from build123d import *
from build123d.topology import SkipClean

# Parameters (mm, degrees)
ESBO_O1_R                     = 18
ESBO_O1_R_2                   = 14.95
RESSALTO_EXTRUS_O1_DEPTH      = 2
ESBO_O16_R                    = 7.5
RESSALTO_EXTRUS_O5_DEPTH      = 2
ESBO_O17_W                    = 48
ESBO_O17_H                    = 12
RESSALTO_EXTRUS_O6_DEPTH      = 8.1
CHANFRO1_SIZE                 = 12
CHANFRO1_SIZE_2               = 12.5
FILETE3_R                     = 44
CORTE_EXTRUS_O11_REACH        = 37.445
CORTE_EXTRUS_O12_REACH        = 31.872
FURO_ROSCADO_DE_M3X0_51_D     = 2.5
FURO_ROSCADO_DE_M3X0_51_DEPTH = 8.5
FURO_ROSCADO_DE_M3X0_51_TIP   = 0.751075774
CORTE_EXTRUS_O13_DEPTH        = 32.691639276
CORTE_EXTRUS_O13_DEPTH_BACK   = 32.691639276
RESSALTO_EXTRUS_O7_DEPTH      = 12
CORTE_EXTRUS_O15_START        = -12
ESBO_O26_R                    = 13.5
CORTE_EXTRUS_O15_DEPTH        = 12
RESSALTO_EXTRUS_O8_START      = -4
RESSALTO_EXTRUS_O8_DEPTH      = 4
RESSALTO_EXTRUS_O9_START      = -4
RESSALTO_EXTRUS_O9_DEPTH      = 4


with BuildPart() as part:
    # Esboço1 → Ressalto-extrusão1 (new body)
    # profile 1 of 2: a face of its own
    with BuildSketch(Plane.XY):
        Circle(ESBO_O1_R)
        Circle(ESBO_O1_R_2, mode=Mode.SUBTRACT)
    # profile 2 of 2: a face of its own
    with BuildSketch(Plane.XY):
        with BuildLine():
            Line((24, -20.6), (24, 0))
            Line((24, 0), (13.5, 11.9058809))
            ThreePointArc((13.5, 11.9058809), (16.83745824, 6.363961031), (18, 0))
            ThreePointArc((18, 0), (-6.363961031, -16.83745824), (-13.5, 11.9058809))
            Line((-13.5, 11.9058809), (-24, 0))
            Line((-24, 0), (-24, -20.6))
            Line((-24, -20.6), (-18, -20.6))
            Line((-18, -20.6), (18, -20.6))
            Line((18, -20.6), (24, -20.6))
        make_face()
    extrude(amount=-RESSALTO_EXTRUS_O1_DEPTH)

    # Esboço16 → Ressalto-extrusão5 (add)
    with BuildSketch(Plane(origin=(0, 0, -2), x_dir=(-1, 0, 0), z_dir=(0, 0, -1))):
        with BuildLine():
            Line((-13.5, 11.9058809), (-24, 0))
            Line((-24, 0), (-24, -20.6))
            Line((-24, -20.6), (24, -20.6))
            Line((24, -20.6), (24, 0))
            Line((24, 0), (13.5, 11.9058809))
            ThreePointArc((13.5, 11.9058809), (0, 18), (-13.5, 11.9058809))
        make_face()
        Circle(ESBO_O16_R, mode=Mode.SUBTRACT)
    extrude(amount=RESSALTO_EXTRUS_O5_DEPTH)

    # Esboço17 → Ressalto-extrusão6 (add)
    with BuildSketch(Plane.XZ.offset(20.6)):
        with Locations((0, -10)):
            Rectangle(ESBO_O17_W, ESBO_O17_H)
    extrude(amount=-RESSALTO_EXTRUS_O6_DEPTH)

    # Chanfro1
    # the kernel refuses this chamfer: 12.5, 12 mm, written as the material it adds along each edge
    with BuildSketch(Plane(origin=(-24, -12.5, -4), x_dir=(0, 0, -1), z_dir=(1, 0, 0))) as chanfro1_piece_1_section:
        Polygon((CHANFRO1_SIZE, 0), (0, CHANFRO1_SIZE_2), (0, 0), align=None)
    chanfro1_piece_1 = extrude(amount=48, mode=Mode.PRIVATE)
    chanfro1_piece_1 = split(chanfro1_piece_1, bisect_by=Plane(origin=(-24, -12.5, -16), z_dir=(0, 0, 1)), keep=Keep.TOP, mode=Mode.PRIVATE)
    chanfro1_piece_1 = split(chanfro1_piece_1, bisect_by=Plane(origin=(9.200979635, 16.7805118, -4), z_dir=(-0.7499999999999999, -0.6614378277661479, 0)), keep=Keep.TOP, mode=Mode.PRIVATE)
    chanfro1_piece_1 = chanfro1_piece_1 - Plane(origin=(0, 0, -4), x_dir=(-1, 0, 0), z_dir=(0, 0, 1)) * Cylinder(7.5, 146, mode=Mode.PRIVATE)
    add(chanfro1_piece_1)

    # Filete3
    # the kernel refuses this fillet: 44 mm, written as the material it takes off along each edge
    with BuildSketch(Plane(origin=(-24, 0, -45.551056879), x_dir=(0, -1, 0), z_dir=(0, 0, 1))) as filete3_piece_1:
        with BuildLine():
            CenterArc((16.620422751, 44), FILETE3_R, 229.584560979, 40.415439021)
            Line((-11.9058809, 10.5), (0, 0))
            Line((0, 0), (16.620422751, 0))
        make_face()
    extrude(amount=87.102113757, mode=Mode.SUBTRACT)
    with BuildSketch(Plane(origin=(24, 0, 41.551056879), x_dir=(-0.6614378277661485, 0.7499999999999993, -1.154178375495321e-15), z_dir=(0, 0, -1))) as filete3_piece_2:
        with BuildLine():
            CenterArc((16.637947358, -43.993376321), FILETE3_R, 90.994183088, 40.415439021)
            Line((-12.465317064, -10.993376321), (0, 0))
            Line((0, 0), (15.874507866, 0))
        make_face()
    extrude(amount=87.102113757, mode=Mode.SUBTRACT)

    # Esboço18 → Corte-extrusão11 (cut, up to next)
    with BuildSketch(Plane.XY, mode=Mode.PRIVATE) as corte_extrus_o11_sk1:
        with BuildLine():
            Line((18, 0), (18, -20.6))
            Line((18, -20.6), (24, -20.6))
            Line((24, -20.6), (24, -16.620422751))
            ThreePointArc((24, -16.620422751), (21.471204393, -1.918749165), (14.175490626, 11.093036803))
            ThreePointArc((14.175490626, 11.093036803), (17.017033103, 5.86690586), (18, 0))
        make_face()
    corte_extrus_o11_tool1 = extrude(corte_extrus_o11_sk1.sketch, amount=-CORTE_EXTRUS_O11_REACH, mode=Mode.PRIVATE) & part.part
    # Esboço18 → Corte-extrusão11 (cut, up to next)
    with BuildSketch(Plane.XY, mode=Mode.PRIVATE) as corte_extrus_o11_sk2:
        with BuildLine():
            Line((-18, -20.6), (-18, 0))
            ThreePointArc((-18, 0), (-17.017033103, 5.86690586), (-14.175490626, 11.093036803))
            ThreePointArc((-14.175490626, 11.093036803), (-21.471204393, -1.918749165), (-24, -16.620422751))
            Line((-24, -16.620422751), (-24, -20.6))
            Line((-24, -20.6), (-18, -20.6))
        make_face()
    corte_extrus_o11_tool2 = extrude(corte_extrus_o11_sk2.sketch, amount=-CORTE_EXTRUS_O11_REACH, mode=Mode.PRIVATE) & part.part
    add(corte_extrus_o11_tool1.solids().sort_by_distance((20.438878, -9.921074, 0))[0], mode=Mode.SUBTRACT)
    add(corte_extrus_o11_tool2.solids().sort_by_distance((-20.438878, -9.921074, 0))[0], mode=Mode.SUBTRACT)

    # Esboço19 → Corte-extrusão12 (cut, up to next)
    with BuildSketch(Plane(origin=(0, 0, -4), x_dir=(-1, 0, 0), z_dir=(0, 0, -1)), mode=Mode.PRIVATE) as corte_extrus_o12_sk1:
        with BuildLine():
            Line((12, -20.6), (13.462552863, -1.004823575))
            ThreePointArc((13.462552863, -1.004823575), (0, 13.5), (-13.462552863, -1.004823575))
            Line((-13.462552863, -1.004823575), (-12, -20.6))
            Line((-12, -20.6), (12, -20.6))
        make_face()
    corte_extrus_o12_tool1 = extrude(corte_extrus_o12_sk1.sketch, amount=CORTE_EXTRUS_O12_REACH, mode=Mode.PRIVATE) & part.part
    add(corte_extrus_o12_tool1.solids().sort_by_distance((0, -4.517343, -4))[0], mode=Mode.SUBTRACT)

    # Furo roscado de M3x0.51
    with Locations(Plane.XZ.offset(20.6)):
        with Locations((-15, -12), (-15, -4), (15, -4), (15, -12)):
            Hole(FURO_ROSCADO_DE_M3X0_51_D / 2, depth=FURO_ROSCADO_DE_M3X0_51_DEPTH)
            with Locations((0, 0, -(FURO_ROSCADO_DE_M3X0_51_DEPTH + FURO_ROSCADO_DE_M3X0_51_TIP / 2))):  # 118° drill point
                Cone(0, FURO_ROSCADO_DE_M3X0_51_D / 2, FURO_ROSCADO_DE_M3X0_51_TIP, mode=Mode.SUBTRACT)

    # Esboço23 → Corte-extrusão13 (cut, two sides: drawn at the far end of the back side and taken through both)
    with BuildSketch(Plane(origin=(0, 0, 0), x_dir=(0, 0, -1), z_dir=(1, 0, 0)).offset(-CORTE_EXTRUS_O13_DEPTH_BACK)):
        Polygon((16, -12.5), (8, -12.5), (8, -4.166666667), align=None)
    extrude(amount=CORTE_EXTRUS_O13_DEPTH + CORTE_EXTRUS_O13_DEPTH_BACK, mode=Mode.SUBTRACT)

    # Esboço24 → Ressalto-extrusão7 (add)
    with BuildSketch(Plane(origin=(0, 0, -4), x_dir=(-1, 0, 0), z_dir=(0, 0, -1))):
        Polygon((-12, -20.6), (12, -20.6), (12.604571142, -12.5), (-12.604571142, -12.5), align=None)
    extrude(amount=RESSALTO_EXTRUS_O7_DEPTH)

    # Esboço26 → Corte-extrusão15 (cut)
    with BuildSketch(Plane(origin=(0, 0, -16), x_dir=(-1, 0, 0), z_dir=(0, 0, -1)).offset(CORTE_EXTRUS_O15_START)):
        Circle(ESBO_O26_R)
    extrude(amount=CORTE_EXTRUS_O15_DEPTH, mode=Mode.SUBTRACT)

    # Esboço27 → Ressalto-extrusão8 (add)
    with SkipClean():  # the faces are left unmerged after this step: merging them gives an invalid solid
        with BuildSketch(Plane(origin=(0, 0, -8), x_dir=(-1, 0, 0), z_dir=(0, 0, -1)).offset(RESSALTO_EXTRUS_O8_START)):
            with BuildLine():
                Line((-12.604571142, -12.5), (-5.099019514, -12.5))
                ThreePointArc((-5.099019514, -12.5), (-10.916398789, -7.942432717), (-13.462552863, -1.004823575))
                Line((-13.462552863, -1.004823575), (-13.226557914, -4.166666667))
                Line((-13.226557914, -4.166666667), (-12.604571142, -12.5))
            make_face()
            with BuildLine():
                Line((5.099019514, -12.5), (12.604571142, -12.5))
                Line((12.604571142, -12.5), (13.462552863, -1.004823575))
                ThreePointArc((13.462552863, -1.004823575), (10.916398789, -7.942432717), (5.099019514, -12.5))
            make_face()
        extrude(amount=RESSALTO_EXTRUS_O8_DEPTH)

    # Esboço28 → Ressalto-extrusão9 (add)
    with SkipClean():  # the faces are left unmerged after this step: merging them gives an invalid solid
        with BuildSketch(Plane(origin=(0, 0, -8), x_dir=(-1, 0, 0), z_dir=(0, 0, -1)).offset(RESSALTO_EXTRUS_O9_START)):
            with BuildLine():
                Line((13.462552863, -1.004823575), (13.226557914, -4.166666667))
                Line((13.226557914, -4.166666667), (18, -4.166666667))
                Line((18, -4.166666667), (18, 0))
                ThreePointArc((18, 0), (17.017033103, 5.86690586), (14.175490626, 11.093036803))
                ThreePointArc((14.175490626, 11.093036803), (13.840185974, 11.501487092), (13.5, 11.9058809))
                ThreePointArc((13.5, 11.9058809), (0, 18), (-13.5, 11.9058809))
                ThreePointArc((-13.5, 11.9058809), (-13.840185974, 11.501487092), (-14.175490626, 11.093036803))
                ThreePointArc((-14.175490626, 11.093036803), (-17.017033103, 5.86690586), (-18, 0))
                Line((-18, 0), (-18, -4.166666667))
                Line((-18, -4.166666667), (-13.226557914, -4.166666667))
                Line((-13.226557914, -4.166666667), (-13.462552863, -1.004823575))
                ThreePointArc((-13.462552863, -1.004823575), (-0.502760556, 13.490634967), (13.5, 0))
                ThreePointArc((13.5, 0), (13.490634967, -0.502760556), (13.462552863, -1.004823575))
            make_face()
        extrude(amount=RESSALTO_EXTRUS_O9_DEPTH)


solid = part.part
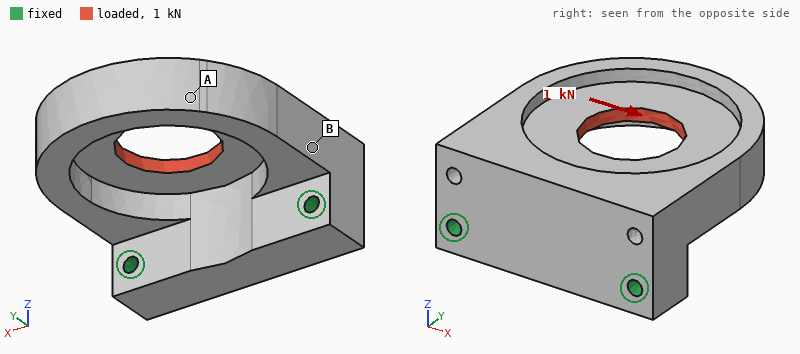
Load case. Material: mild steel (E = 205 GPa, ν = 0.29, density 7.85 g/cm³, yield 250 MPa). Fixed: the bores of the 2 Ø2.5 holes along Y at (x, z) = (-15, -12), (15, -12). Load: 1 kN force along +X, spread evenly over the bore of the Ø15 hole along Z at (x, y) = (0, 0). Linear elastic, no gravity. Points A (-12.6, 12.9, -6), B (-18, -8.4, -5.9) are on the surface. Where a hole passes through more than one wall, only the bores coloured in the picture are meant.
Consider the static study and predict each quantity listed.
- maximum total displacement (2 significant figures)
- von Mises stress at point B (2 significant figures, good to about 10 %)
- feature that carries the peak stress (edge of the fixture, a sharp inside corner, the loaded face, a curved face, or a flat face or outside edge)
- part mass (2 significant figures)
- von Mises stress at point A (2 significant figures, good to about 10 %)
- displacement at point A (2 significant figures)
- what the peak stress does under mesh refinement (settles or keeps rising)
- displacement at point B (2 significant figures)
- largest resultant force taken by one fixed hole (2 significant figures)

9.7 µm
22 MPa
edge of the fixture
63 g
7.1 MPa
9.3 µm
keeps rising
3.1 µm
760 N
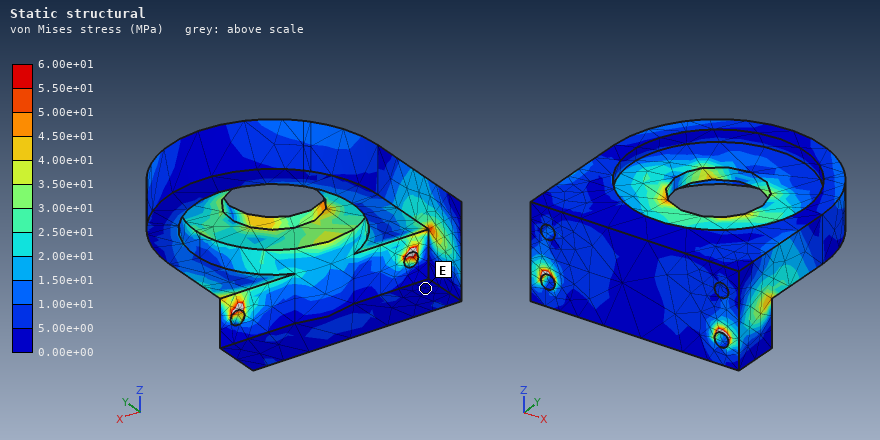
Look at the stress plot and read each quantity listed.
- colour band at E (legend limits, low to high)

0.00e+00 to 5.00e+00 MPa
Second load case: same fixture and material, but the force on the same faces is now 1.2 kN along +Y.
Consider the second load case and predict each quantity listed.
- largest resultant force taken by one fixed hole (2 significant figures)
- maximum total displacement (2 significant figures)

600 N
17 µm
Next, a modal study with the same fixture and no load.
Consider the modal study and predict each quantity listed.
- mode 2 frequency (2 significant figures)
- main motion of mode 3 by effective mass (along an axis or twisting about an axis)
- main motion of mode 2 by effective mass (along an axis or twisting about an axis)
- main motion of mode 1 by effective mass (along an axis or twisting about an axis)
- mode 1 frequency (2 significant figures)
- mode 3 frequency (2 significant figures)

8800 Hz
along X
along X
along Z
4100 Hz
12 kHz
